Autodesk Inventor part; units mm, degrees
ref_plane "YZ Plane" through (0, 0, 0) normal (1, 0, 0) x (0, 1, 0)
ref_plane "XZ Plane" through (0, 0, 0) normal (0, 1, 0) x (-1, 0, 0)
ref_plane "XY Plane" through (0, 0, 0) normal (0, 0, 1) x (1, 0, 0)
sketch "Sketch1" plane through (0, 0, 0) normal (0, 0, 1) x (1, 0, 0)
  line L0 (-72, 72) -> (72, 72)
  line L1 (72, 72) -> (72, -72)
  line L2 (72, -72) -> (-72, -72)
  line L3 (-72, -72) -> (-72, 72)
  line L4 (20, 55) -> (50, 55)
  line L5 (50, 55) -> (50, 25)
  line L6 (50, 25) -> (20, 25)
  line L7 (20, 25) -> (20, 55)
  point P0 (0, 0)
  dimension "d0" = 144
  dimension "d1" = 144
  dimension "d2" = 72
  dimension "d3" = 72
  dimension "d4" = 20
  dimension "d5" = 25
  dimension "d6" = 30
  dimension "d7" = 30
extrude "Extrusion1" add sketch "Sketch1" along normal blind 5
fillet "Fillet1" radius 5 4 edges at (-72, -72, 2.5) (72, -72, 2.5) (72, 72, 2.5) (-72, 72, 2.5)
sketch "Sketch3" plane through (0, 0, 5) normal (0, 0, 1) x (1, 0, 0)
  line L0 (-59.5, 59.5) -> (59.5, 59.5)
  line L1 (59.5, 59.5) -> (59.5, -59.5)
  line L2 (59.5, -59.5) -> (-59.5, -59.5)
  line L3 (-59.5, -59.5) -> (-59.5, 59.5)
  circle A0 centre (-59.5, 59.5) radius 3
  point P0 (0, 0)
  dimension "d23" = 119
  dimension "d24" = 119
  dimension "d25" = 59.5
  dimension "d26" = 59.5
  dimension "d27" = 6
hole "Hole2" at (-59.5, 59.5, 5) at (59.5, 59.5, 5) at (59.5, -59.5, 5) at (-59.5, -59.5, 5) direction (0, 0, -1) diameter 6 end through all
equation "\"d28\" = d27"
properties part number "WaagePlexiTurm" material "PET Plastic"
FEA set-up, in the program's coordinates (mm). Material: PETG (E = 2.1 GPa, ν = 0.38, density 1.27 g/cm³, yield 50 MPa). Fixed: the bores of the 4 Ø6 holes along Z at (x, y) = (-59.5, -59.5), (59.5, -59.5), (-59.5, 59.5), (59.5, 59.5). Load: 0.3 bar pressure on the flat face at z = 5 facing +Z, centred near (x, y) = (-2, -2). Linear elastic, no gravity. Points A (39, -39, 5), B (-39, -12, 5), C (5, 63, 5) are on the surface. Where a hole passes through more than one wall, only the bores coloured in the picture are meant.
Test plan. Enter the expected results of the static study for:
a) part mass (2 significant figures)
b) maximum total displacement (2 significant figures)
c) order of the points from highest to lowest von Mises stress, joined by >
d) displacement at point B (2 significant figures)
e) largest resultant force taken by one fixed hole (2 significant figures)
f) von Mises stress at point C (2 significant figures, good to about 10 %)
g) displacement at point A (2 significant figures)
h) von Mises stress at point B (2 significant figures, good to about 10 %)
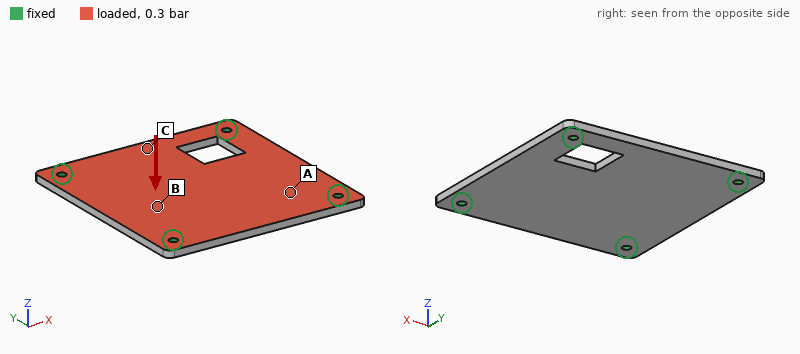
130 g
1.9 mm
C > B > A
1.3 mm
160 N
5.9 MPa
0.83 mm
4.5 MPa
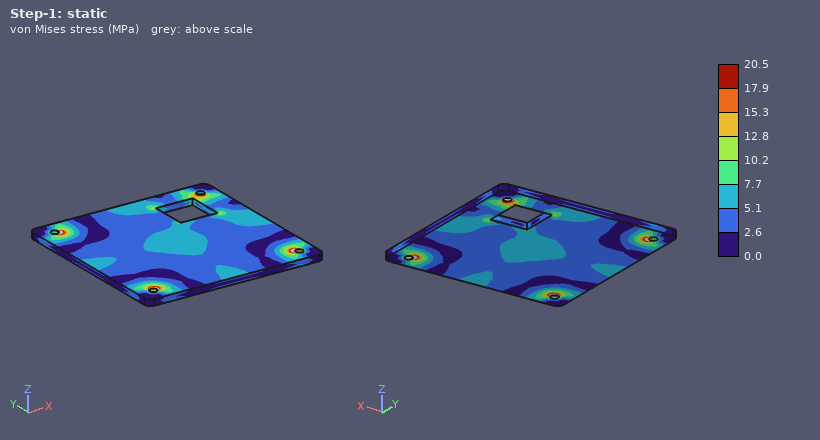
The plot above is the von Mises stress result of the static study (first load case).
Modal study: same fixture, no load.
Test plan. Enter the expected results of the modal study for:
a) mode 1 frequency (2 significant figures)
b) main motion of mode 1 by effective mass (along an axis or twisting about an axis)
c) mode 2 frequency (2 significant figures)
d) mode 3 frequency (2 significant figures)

300 Hz
along Z
490 Hz
510 Hz
